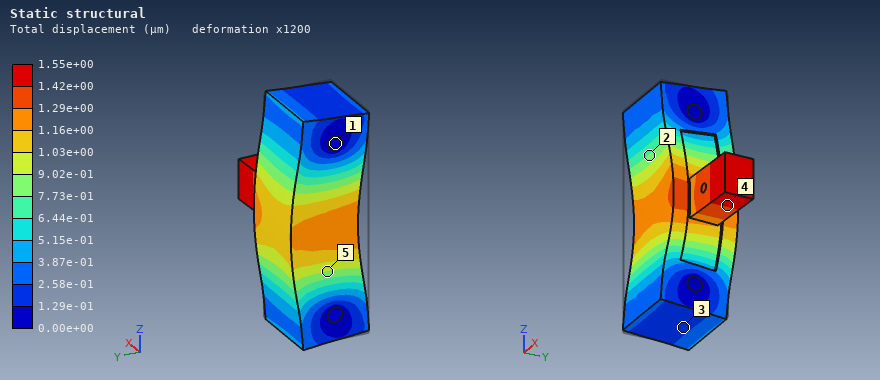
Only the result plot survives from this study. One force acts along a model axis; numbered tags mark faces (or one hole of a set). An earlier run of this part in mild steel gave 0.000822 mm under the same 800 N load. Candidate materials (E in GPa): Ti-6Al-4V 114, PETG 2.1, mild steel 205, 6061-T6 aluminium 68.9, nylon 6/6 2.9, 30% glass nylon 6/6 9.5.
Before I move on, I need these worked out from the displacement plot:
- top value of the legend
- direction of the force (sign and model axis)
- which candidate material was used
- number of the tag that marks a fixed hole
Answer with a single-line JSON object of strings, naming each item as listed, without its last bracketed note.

{"top value of the legend": "1.55e+00 µm", "direction of the force": "+Y", "which candidate material was used": "Ti-6Al-4V", "number of the tag that marks a fixed hole": "1"}
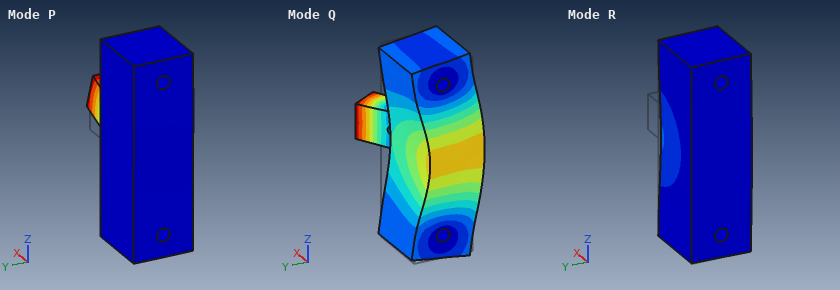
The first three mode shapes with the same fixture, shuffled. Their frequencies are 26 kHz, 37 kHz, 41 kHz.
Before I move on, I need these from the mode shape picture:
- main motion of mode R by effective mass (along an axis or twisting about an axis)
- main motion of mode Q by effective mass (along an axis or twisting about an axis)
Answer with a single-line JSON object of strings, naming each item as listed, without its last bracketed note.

{"main motion of mode R by effective mass": "along Y", "main motion of mode Q by effective mass": "along Y"}
